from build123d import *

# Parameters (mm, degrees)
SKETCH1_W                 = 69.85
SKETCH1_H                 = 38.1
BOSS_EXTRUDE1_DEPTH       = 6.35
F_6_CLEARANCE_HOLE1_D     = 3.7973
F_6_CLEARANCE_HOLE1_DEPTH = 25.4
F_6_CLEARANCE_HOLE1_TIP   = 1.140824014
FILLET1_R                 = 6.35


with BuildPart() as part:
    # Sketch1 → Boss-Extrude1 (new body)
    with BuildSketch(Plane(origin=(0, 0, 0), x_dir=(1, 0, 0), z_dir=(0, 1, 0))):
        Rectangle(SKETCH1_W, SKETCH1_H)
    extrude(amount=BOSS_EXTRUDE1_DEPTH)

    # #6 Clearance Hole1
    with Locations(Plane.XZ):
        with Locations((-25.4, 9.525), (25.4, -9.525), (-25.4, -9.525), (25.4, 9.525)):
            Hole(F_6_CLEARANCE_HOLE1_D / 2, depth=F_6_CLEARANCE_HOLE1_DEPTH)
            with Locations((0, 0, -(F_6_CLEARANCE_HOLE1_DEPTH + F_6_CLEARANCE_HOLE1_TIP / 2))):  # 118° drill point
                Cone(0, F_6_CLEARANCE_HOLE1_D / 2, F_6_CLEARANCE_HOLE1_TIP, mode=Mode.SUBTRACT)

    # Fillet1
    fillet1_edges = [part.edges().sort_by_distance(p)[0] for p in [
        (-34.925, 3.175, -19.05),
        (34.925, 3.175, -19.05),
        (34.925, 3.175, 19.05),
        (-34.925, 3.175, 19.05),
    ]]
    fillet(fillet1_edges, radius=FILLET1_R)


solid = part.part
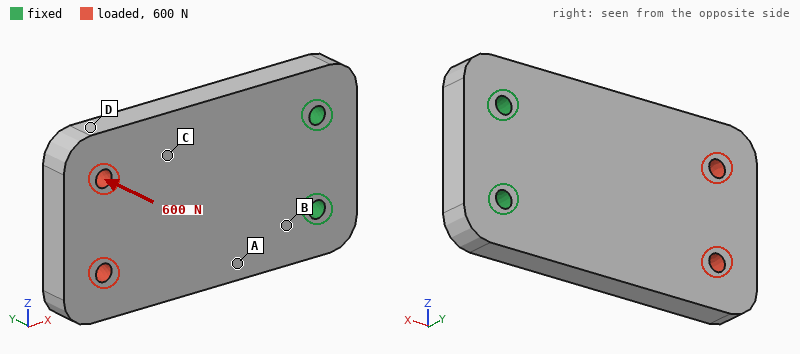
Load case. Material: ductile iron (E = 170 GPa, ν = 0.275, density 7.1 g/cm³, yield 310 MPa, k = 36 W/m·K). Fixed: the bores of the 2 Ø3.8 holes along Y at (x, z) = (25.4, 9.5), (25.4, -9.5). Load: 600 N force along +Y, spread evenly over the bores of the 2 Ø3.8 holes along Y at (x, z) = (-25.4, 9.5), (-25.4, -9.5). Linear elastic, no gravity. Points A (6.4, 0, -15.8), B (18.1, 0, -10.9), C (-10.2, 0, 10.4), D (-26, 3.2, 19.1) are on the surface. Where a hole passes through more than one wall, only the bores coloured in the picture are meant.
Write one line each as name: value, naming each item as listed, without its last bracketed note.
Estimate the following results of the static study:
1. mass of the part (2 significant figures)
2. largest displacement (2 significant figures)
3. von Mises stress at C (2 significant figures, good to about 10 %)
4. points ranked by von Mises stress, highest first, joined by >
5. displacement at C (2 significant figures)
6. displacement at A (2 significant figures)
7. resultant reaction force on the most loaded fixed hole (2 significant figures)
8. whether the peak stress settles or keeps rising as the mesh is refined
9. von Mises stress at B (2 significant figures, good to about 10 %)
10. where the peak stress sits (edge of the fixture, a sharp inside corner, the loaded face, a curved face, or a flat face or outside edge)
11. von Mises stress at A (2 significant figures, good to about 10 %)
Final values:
mass of the part: 120 g
largest displacement: 0.25 mm
von Mises stress at C: 36 MPa
points ranked by von Mises stress, highest first, joined by >: B > A > C > D
displacement at C: 0.11 mm
displacement at A: 0.039 mm
resultant reaction force on the most loaded fixed hole: 300 N
whether the peak stress settles or keeps rising as the mesh is refined: keeps rising
von Mises stress at B: 100 MPa
where the peak stress sits: edge of the fixture
von Mises stress at A: 74 MPa
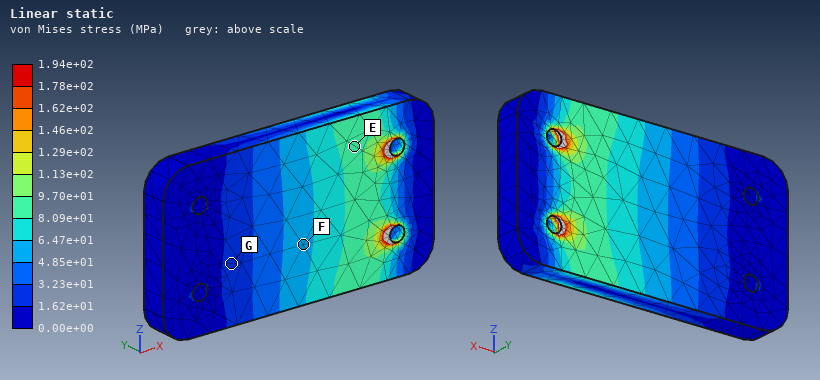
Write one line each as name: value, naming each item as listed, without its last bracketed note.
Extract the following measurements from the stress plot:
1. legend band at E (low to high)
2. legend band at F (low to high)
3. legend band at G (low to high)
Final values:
legend band at E: 8.09e+01 to 9.70e+01 MPa
legend band at F: 4.85e+01 to 6.47e+01 MPa
legend band at G: 1.62e+01 to 3.23e+01 MPa
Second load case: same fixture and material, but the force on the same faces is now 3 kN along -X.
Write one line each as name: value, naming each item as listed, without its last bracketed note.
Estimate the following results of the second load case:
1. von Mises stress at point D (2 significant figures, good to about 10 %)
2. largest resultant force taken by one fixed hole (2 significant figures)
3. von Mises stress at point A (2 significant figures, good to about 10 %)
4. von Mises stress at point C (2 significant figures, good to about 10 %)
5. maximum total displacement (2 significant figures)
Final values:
von Mises stress at point D: 3.3 MPa
largest resultant force taken by one fixed hole: 1.5 kN
von Mises stress at point A: 12 MPa
von Mises stress at point C: 13 MPa
maximum total displacement: 4.6 µm
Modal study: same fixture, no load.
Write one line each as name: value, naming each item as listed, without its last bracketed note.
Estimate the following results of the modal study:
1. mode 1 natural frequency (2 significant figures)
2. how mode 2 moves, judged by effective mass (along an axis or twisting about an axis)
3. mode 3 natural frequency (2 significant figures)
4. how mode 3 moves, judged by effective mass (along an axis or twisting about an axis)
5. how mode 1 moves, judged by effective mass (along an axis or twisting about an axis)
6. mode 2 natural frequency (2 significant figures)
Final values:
mode 1 natural frequency: 1400 Hz
how mode 2 moves, judged by effective mass: twisting about X
mode 3 natural frequency: 5800 Hz
how mode 3 moves, judged by effective mass: along Z
how mode 1 moves, judged by effective mass: along Y
mode 2 natural frequency: 4600 Hz
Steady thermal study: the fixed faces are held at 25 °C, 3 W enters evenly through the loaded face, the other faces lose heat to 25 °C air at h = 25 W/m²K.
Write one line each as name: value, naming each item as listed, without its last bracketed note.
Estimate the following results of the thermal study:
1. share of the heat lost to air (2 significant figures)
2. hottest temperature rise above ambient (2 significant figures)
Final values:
share of the heat lost to air: 35 %
hottest temperature rise above ambient: 14 K
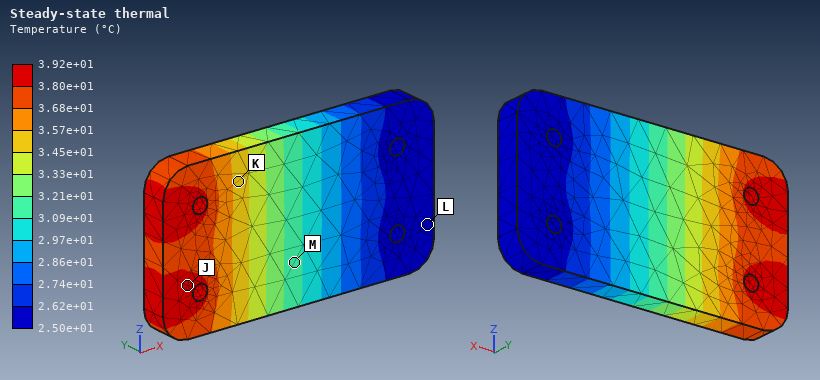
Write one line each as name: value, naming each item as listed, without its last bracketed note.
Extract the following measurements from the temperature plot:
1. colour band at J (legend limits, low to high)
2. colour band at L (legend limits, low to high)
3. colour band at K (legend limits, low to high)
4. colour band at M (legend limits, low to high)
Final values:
colour band at J: 3.80e+01 to 3.92e+01 °C
colour band at L: 2.50e+01 to 2.62e+01 °C
colour band at K: 3.45e+01 to 3.57e+01 °C
colour band at M: 3.09e+01 to 3.21e+01 °C
